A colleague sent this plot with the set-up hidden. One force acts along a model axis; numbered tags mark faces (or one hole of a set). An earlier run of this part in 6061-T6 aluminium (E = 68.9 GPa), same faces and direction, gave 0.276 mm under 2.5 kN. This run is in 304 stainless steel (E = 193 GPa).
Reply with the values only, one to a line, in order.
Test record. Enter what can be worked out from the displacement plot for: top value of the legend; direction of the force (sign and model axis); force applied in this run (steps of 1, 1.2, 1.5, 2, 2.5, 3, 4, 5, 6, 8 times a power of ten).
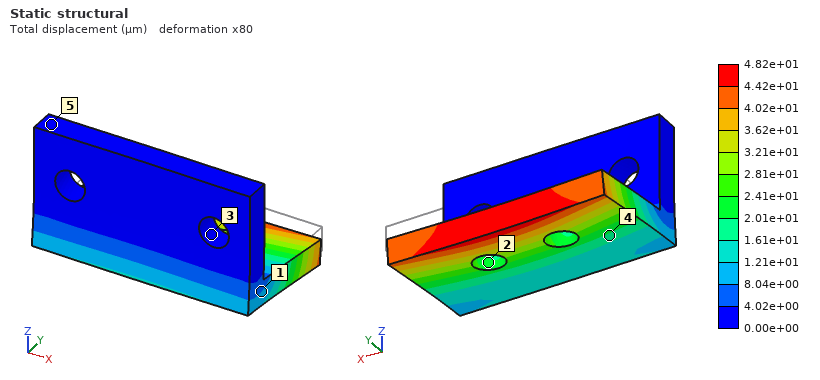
4.82e+01 µm
-Z
1.2 kN
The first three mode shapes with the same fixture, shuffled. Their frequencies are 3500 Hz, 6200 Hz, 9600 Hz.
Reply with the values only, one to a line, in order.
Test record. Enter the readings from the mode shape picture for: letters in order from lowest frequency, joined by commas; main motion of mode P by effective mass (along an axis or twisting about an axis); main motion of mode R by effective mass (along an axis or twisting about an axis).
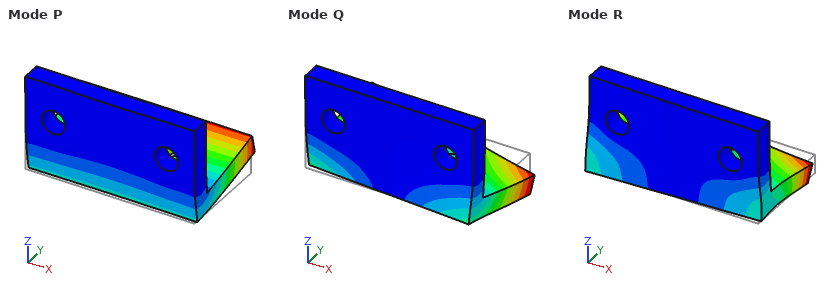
P, Q, R
along Z
along X
